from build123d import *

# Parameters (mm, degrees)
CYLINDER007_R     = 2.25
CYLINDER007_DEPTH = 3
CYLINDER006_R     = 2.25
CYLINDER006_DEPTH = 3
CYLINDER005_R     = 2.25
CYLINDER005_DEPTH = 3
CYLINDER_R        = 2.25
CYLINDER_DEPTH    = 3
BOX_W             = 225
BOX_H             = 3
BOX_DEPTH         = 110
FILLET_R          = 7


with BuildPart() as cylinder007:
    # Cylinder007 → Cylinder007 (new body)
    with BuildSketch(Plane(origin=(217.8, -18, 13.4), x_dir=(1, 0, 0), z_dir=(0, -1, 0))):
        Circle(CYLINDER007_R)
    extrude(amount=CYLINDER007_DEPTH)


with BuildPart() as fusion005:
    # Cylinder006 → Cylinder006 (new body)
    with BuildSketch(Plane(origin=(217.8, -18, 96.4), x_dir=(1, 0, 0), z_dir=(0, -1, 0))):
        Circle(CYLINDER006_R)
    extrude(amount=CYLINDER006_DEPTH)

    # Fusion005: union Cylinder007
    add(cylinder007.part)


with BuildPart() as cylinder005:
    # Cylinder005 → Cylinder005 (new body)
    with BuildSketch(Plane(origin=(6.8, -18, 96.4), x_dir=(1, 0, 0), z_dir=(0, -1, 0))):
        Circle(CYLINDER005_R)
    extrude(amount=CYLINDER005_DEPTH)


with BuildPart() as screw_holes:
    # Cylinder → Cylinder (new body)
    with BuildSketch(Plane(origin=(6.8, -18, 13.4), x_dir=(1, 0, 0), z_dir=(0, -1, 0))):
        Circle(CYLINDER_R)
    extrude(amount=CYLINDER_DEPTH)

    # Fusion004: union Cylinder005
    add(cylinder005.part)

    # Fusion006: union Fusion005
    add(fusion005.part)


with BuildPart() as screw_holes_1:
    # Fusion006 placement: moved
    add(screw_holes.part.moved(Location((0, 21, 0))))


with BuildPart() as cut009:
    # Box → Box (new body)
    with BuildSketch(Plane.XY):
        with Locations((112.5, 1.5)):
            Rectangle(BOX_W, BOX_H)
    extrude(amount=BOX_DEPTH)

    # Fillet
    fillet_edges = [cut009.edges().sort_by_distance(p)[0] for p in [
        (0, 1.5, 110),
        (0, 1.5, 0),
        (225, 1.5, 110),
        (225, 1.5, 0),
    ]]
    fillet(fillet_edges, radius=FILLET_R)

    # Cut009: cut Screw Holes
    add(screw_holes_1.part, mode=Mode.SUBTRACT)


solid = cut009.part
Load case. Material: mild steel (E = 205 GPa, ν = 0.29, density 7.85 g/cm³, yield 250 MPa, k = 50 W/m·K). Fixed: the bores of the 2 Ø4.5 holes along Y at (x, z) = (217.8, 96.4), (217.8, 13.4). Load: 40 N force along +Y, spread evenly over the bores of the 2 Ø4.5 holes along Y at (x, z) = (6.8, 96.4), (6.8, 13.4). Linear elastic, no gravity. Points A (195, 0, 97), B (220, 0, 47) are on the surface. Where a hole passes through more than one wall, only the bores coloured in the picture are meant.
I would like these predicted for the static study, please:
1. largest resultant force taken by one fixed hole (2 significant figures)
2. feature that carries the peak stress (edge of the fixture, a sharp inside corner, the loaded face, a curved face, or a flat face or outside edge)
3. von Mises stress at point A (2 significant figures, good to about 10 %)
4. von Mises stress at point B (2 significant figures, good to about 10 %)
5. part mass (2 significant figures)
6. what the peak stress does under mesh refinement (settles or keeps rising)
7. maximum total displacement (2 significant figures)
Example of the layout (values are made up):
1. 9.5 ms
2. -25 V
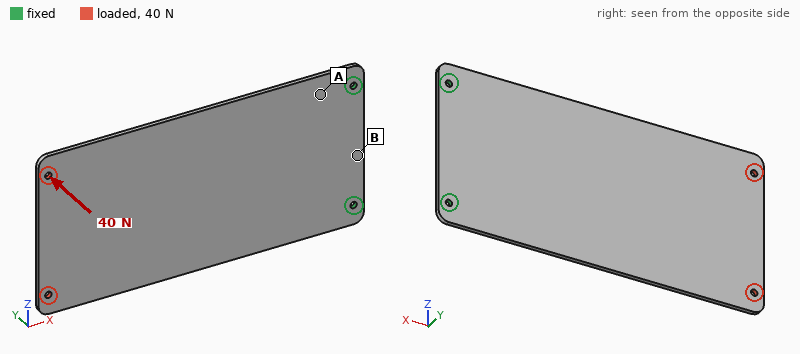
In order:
1. 20 N
2. edge of the fixture
3. 49 MPa
4. 15 MPa
5. 580 g
6. keeps rising
7. 2.9 mm
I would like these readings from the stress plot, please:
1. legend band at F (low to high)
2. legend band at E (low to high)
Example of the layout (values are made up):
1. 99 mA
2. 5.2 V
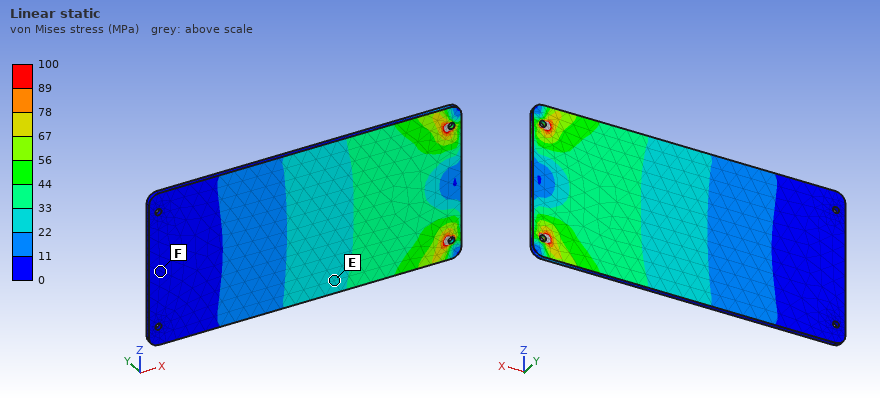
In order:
1. 0 to 11 MPa
2. 22 to 33 MPa
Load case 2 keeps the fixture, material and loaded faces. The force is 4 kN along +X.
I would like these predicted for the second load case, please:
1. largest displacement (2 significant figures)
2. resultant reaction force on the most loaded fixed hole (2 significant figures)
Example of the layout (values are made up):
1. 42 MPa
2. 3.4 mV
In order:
1. 19 µm
2. 2.0 kN
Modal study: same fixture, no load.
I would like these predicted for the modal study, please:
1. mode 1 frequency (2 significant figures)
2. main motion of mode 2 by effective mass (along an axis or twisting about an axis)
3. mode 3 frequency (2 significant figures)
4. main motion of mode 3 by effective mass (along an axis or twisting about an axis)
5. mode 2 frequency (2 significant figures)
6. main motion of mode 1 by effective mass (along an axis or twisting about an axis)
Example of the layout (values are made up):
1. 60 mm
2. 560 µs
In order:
1. 49 Hz
2. twisting about X
3. 310 Hz
4. along Y
5. 230 Hz
6. along Y
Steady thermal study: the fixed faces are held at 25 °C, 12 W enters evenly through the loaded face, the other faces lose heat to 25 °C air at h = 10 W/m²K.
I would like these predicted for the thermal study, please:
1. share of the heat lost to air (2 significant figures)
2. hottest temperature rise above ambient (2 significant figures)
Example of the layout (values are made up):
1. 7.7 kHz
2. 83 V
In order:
1. 88 %
2. 74 K
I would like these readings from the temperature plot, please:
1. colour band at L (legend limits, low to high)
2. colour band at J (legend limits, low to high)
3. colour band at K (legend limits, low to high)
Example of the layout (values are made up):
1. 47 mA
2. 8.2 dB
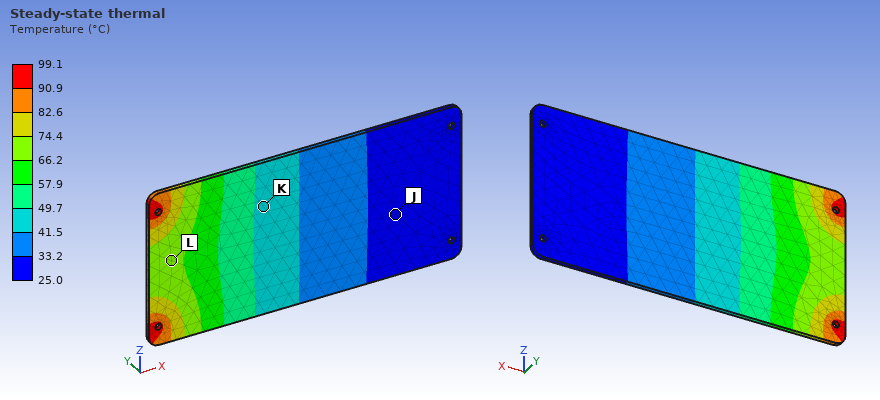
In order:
1. 66.2 to 74.4 °C
2. 25.0 to 33.2 °C
3. 41.5 to 49.7 °C
